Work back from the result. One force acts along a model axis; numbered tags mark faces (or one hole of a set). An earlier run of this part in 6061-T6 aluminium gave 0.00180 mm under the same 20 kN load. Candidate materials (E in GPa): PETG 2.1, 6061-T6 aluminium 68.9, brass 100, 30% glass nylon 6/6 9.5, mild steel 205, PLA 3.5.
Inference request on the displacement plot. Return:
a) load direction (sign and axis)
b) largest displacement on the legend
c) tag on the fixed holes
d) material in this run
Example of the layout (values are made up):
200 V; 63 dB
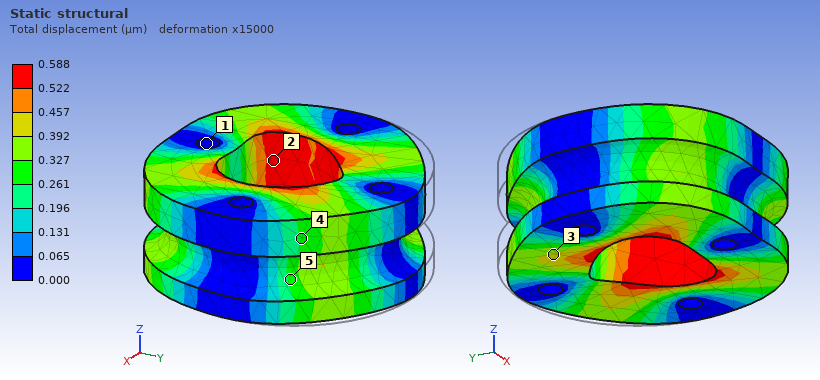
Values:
-Y; 0.588 µm; 1; mild steel
